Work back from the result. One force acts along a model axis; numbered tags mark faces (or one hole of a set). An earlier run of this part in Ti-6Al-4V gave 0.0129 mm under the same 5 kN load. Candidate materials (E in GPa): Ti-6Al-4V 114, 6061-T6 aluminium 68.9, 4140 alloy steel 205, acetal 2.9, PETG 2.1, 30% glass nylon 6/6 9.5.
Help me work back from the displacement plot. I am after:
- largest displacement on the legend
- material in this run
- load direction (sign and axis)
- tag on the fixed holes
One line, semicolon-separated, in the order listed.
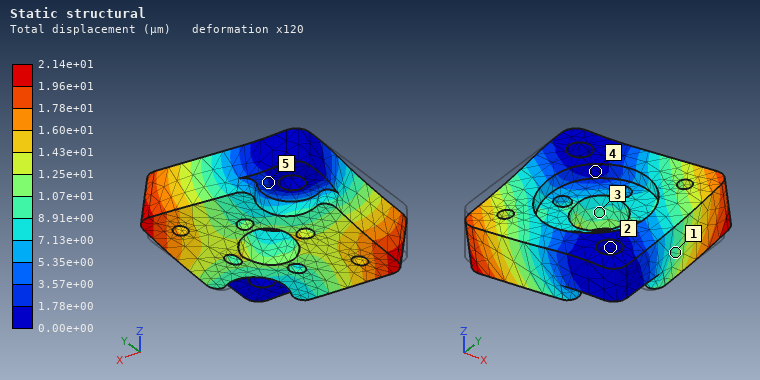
2.14e+01 µm; 6061-T6 aluminium; +X; 2
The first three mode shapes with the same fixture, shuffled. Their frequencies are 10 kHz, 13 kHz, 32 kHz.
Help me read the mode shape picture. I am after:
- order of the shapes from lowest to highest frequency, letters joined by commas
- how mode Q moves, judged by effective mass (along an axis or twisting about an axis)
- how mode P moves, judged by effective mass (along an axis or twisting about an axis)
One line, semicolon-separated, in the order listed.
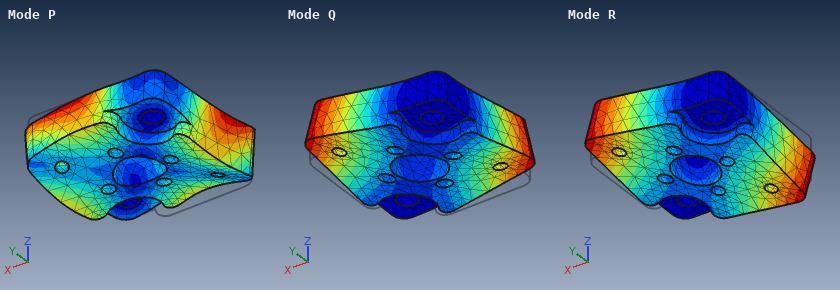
R, Q, P; along Z; twisting about Z
